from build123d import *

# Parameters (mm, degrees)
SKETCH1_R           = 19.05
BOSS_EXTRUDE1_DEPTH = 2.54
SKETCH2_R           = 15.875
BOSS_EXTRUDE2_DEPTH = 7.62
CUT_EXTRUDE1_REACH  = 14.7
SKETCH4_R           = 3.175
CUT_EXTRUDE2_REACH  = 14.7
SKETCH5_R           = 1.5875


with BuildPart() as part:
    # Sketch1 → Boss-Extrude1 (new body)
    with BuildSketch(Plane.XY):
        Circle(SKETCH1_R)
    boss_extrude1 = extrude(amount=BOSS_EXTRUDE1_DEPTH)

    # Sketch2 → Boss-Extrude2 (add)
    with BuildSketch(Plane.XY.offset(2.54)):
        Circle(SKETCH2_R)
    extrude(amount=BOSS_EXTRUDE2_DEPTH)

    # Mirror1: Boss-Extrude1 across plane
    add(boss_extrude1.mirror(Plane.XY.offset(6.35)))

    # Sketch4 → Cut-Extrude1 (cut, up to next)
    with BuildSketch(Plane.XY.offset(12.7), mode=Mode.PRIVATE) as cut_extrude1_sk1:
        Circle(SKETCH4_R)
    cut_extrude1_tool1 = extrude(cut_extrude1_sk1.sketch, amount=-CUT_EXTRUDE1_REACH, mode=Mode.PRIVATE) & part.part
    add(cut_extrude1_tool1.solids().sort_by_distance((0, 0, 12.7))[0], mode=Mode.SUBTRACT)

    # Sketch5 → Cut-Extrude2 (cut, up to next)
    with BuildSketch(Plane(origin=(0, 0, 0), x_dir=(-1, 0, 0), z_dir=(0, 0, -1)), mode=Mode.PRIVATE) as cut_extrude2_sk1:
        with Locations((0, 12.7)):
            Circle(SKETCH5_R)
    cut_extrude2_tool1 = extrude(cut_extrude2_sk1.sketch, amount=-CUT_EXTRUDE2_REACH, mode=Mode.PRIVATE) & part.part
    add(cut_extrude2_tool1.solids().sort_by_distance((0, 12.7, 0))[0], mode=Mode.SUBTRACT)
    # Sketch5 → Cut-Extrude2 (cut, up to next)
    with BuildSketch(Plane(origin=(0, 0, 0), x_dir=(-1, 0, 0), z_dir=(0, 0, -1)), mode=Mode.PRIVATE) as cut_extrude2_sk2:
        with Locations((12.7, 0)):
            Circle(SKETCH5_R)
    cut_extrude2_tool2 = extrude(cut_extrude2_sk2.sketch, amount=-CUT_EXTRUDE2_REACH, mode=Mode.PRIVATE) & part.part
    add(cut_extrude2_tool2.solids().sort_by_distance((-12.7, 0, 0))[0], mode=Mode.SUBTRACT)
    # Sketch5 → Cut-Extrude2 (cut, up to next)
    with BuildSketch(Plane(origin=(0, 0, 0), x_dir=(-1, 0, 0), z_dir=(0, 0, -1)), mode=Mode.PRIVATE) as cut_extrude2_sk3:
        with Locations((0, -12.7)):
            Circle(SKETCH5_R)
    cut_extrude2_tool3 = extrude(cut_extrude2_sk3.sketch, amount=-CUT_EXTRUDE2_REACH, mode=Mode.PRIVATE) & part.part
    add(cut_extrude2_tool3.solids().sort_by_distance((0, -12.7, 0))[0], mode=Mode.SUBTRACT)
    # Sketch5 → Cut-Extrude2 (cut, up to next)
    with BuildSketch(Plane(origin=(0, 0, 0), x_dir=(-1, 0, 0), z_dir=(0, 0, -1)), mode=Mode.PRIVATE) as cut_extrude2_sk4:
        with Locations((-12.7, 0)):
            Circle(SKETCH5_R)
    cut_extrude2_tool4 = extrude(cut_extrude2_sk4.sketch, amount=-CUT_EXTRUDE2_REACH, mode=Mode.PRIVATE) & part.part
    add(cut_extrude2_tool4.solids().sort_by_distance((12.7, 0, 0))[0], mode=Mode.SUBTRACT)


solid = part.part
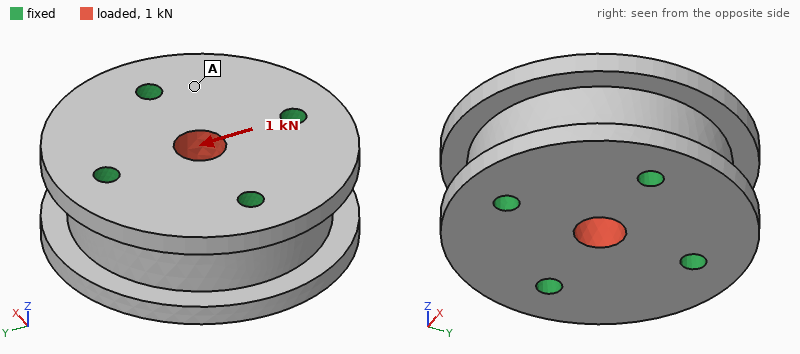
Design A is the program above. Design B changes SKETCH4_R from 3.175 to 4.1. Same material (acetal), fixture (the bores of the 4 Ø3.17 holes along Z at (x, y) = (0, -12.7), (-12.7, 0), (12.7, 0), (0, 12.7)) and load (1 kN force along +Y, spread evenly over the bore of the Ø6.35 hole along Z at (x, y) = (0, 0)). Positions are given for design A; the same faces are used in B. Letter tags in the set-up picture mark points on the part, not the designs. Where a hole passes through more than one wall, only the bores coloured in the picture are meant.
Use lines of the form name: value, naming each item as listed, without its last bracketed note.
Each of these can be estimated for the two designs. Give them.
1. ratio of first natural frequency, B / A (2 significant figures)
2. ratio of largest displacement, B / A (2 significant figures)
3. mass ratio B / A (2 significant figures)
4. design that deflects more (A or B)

ratio of first natural frequency, B / A: 0.99
ratio of largest displacement, B / A: 0.88
mass ratio B / A: 0.98
design that deflects more: A
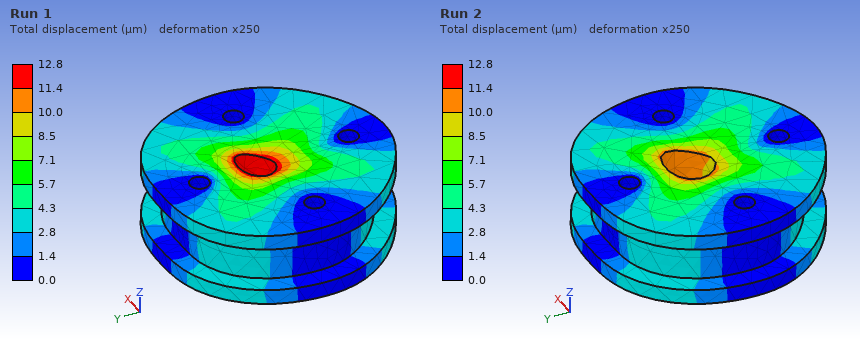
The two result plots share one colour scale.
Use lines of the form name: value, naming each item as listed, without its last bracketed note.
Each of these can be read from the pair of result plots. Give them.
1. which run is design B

which run is design B: Run 2
